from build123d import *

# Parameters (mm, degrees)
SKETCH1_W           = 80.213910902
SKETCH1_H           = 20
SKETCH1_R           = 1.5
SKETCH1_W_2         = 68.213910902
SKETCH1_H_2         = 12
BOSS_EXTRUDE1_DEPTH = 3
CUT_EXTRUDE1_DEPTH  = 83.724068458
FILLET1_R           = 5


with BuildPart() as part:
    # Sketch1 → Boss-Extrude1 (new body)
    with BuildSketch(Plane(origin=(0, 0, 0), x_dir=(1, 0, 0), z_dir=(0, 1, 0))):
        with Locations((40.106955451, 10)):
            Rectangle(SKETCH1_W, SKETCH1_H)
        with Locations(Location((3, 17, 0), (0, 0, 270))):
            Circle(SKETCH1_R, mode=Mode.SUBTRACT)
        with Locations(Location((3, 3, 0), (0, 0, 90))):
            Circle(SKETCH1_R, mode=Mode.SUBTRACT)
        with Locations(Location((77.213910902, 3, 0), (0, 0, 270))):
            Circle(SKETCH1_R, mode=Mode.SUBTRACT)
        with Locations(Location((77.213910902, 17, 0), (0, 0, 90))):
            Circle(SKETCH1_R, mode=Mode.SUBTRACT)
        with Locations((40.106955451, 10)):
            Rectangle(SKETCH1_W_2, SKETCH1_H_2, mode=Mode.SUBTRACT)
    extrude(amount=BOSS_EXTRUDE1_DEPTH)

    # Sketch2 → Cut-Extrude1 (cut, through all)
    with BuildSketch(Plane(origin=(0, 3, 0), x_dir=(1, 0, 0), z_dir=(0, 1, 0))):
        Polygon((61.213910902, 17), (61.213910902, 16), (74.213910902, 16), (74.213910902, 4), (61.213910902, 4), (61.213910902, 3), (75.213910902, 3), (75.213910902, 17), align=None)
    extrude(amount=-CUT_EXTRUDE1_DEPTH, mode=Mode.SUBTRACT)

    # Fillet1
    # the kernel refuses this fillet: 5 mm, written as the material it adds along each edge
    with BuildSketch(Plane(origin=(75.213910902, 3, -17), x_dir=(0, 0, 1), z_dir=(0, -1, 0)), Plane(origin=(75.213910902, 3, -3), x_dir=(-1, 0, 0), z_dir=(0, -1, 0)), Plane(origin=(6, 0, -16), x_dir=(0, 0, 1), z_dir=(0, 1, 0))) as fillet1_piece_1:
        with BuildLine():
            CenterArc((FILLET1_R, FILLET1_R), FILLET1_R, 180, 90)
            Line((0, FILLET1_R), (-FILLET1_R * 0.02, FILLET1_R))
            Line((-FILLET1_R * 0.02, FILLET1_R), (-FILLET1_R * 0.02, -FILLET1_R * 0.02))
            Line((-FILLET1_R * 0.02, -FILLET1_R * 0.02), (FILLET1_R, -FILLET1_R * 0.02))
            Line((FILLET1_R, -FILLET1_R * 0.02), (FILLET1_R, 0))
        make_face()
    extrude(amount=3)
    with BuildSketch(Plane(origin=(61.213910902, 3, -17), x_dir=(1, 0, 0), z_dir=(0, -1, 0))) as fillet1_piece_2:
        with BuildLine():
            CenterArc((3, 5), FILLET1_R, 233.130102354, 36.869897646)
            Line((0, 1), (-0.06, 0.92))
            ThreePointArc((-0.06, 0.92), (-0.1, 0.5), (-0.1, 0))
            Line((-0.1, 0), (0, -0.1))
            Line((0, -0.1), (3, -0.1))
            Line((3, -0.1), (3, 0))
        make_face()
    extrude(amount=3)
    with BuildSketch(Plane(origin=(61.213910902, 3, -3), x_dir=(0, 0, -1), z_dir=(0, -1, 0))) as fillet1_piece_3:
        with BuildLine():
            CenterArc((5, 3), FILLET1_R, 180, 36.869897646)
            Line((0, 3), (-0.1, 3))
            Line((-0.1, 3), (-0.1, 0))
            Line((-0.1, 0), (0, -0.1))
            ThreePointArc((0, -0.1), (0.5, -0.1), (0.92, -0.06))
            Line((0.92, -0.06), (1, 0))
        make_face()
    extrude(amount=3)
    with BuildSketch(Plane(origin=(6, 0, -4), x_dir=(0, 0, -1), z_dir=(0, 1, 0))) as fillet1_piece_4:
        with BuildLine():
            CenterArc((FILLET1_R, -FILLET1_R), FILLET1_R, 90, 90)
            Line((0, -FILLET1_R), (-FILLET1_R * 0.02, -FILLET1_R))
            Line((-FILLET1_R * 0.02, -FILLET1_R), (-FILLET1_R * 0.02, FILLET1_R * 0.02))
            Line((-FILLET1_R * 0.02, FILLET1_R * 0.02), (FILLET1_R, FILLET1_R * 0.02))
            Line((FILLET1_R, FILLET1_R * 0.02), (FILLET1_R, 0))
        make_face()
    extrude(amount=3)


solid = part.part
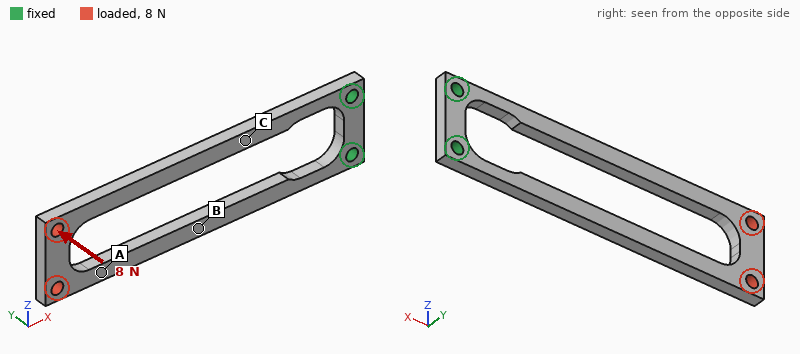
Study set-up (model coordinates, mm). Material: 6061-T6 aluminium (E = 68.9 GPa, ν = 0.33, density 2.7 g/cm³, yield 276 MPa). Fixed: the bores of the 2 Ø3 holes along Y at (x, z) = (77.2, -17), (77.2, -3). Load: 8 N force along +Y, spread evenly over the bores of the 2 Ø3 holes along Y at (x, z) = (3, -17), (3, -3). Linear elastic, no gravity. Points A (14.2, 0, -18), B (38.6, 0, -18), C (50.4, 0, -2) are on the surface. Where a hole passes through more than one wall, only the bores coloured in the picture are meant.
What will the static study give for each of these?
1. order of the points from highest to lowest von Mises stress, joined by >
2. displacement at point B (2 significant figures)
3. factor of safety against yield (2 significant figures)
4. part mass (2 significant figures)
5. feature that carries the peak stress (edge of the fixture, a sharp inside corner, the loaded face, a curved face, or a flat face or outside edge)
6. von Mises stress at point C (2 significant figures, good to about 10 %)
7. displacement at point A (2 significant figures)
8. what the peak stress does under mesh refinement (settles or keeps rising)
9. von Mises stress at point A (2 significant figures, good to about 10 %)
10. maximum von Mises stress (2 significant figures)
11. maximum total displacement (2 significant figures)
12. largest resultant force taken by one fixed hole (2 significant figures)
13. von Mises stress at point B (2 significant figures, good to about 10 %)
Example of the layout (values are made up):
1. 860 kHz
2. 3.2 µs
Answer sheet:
1. C > B > A
2. 0.31 mm
3. 4.1
4. 6.0 g
5. a curved face
6. 32 MPa
7. 0.72 mm
8. settles
9. 7.5 MPa
10. 67 MPa
11. 0.98 mm
12. 4.0 N
13. 24 MPa
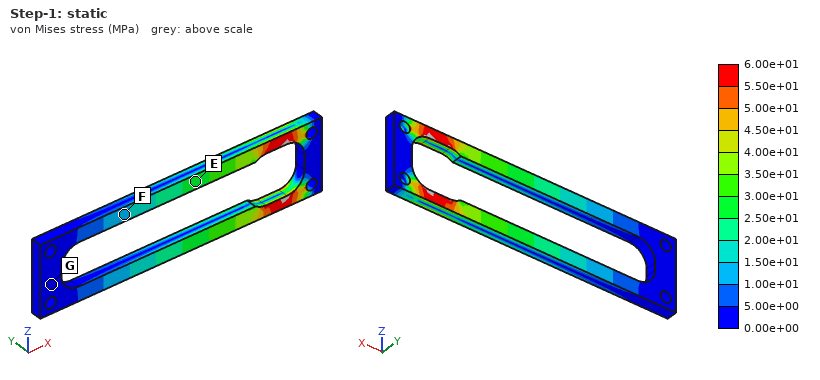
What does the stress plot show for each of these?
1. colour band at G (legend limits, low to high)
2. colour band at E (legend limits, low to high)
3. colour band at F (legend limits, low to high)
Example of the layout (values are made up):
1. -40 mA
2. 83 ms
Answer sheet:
1. 0.00e+00 to 5.00e+00 MPa
2. 2.50e+01 to 3.00e+01 MPa
3. 1.00e+01 to 1.50e+01 MPa
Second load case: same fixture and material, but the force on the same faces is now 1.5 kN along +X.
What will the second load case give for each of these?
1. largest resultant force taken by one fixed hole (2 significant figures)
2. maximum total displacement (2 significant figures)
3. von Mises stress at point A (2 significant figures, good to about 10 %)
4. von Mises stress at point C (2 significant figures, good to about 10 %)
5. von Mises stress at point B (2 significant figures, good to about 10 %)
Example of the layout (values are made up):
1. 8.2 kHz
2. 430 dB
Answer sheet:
1. 750 N
2. 77 µm
3. 63 MPa
4. 63 MPa
5. 63 MPa
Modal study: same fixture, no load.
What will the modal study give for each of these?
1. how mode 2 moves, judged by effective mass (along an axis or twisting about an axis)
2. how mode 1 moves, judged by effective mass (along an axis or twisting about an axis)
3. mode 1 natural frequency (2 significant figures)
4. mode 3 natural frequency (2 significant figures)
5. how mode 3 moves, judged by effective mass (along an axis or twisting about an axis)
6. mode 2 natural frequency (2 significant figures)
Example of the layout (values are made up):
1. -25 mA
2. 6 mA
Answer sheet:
1. along Z
2. along Y
3. 340 Hz
4. 1600 Hz
5. twisting about X
6. 750 Hz
